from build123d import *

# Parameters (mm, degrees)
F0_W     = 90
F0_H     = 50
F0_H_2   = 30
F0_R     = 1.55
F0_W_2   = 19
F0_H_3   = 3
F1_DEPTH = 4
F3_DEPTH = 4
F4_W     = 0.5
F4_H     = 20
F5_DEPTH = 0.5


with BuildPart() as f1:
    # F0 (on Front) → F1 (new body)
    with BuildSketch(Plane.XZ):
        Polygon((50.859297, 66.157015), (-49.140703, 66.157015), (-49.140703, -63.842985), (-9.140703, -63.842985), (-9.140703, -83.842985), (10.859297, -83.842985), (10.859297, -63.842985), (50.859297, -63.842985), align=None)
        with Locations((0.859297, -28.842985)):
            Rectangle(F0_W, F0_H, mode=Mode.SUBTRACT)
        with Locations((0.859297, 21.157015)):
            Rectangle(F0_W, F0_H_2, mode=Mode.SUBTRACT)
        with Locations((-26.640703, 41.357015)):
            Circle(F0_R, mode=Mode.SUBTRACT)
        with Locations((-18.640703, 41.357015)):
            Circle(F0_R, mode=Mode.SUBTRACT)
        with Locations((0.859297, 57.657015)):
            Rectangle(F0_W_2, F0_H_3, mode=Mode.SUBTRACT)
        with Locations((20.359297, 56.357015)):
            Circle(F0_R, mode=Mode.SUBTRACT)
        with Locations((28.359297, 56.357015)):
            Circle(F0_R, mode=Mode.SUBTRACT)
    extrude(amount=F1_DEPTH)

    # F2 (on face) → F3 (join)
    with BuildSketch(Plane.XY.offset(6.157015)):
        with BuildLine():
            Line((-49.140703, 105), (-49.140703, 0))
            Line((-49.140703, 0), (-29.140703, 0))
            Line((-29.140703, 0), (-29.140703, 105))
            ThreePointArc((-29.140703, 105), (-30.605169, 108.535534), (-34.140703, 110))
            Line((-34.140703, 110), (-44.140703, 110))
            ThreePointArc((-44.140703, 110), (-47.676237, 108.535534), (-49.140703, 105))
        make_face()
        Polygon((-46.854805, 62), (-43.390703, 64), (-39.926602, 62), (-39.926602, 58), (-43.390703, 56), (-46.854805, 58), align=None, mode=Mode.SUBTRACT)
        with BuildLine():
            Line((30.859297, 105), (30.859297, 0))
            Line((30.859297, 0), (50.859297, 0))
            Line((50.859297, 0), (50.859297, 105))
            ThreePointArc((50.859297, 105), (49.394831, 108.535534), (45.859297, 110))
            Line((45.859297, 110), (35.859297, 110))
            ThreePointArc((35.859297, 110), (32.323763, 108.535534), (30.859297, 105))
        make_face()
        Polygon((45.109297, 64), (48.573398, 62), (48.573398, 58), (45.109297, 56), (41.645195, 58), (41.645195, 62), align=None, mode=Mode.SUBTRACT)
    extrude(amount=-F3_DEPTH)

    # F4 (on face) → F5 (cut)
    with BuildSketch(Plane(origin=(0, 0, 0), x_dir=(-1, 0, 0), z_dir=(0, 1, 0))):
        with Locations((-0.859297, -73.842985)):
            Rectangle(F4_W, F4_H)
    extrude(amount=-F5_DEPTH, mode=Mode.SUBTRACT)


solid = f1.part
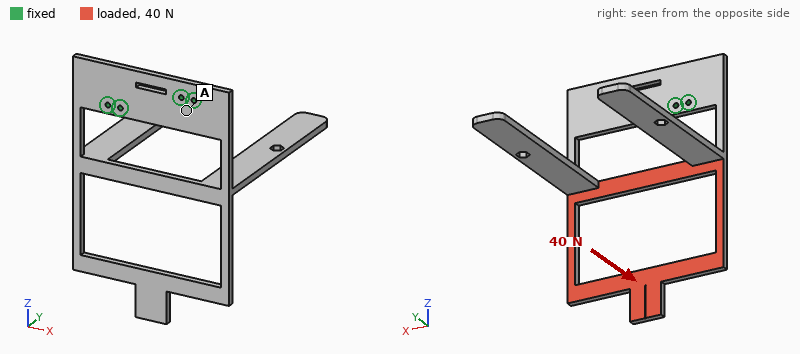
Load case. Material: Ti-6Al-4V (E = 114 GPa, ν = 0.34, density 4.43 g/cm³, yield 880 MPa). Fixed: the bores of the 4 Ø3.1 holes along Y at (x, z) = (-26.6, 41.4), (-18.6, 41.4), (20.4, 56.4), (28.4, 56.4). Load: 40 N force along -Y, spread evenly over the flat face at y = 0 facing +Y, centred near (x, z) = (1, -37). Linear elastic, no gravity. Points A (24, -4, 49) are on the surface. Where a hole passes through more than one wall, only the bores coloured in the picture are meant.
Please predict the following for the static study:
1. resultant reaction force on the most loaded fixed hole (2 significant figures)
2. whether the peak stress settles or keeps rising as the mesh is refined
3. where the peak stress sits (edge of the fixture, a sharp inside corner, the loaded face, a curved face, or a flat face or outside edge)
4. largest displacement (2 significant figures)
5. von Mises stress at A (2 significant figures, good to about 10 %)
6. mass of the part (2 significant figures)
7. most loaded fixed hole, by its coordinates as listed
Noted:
33 N
keeps rising
a sharp inside corner
2.3 mm
16 MPa
180 g
(-26.6, 41.4)
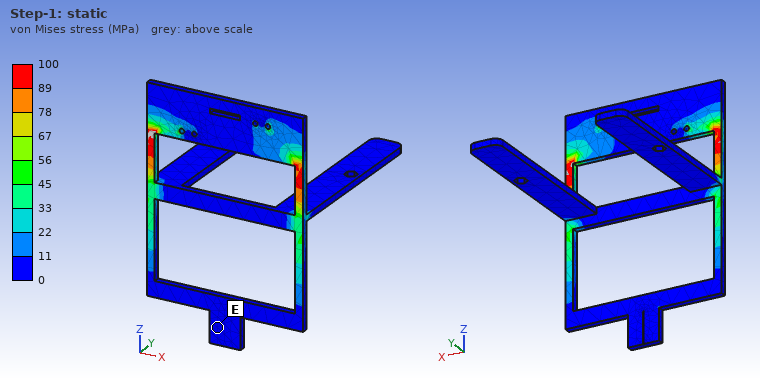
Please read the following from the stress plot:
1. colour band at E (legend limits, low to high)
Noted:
0 to 11 MPa
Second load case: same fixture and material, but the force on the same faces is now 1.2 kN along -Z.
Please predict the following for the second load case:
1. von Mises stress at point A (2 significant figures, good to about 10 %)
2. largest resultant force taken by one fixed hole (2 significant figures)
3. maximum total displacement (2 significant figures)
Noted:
16 MPa
1000 N
2.5 mm
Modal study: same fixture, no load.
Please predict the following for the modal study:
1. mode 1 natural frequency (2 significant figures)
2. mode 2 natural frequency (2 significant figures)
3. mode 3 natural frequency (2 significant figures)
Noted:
78 Hz
160 Hz
200 Hz
